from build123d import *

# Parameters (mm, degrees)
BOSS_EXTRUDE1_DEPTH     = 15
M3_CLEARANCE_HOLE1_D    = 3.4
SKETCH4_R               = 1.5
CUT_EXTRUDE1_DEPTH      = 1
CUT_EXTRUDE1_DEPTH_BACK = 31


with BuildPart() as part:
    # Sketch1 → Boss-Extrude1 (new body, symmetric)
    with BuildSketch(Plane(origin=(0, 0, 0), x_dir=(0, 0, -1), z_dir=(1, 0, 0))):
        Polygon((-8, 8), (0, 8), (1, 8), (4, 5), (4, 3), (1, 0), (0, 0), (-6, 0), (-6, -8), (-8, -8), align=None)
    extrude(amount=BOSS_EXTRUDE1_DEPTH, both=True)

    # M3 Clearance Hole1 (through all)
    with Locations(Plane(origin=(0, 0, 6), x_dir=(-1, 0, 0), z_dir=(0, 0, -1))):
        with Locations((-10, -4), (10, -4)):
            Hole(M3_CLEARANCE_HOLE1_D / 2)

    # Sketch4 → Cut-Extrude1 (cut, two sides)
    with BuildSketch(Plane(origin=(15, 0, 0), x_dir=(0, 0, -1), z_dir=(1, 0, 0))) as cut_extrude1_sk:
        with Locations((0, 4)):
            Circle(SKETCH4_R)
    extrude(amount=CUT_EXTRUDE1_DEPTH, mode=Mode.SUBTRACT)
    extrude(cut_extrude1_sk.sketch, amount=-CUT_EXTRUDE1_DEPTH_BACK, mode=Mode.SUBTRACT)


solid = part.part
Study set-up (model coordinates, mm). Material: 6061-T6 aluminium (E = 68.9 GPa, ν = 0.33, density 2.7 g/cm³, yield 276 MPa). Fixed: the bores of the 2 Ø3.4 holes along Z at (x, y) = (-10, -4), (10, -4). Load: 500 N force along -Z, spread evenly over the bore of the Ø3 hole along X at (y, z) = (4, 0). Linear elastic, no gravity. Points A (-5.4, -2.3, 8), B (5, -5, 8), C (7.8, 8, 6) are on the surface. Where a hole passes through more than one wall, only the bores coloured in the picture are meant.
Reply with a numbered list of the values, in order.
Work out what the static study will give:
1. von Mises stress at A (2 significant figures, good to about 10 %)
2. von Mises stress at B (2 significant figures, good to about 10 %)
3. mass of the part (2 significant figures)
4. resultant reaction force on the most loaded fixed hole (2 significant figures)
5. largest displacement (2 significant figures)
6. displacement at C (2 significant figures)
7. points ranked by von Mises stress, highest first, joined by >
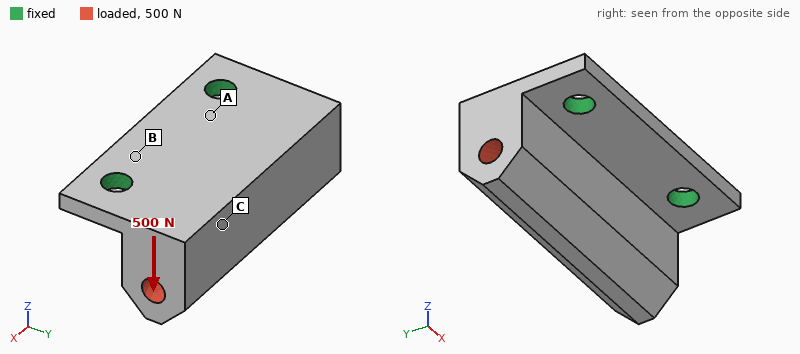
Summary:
1. 85 MPa
2. 43 MPa
3. 7.7 g
4. 250 N
5. 0.11 mm
6. 0.086 mm
7. A > B > C
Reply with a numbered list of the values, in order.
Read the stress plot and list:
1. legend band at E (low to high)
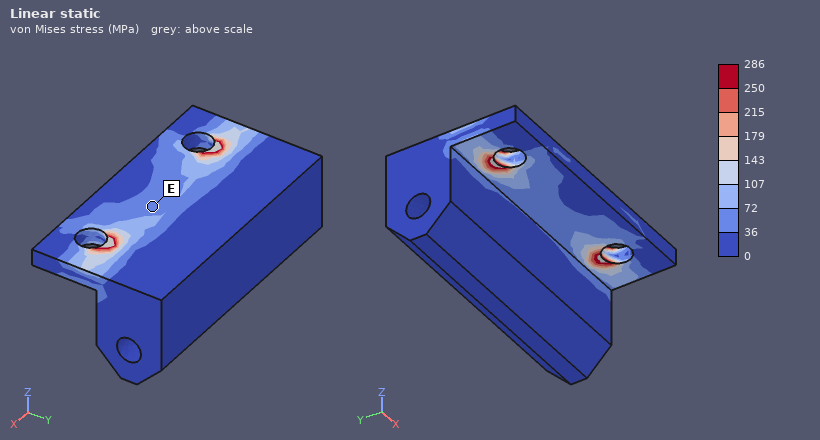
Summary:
1. 36 to 72 MPa
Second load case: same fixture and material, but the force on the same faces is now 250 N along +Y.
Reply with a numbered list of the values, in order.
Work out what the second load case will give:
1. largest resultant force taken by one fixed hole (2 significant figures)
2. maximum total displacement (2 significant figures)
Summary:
1. 130 N
2. 73 µm
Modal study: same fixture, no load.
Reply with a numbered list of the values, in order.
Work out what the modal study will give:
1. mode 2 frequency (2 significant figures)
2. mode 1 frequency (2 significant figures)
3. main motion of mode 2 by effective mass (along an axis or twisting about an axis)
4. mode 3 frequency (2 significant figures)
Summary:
1. 15 kHz
2. 4300 Hz
3. along X
4. 24 kHz
